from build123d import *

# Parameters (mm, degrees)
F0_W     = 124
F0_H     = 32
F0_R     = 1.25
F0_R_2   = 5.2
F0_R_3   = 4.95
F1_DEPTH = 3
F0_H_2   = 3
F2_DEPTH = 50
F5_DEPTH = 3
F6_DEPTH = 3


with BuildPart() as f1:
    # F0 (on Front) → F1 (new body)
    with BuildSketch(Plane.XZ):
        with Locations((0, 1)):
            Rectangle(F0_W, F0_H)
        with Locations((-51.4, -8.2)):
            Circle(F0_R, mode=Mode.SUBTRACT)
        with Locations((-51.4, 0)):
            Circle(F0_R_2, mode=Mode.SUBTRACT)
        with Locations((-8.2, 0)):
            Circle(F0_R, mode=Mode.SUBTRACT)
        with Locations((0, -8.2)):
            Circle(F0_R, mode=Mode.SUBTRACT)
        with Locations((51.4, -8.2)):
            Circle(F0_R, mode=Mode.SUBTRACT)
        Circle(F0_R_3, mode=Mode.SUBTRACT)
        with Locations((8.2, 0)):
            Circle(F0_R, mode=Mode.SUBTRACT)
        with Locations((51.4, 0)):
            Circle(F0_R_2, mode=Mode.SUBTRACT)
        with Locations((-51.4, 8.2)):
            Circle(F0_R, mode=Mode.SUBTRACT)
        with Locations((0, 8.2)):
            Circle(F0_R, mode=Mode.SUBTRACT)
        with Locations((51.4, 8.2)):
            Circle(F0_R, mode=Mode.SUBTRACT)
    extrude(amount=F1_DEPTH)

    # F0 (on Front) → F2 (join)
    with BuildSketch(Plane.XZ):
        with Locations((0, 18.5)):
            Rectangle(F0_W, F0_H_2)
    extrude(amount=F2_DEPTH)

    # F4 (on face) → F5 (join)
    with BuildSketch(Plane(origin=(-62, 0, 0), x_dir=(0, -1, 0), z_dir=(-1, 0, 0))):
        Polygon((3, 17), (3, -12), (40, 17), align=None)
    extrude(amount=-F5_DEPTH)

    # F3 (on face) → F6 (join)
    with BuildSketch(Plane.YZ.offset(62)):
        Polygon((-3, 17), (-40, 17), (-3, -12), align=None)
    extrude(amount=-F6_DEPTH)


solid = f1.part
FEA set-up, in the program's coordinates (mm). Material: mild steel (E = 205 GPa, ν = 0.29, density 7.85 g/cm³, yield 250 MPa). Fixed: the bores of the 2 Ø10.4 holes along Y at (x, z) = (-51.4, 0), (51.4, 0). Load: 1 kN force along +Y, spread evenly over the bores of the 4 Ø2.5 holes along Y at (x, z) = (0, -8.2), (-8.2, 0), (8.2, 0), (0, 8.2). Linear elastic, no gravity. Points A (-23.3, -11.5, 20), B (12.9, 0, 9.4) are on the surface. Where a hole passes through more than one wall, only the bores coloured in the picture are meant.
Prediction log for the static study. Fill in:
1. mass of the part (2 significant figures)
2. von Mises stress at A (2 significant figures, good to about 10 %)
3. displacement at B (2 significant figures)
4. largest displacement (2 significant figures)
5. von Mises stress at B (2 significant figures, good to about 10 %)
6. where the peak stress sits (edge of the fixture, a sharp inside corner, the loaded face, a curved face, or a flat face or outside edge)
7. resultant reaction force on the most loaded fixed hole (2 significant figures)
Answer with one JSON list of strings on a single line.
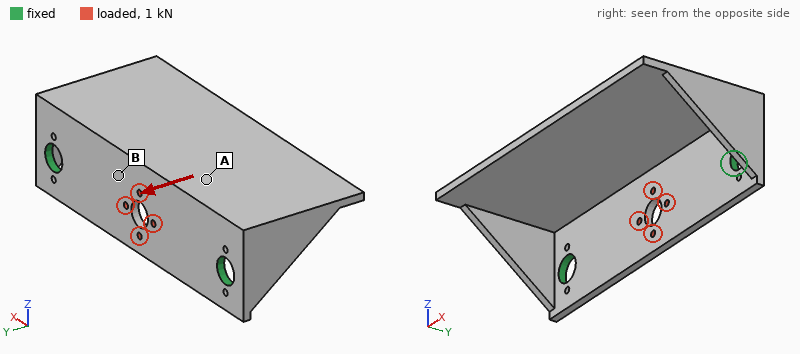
["260 g", "23 MPa", "0.048 mm", "0.19 mm", "81 MPa", "the loaded face", "510 N"]
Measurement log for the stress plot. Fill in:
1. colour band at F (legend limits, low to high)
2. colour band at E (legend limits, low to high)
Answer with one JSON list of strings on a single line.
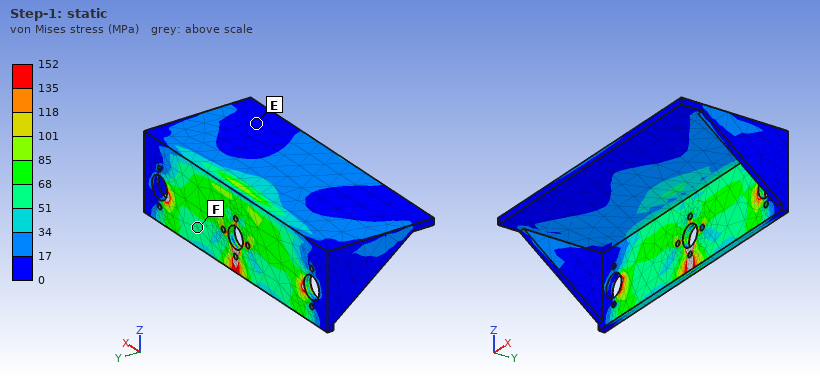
["51 to 68 MPa", "0 to 17 MPa"]
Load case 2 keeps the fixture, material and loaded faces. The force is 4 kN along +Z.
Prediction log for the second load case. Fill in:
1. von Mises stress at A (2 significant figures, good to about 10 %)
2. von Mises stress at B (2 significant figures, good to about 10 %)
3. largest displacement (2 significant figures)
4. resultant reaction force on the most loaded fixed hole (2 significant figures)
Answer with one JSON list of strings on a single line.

["20 MPa", "44 MPa", "28 µm", "2.2 kN"]
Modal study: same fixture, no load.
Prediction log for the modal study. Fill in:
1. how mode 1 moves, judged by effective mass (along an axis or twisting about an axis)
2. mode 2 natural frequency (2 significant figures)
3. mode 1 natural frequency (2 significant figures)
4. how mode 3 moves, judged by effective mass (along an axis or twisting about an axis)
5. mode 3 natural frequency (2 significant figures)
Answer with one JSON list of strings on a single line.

["along Z", "1900 Hz", "1100 Hz", "along Y", "2400 Hz"]
